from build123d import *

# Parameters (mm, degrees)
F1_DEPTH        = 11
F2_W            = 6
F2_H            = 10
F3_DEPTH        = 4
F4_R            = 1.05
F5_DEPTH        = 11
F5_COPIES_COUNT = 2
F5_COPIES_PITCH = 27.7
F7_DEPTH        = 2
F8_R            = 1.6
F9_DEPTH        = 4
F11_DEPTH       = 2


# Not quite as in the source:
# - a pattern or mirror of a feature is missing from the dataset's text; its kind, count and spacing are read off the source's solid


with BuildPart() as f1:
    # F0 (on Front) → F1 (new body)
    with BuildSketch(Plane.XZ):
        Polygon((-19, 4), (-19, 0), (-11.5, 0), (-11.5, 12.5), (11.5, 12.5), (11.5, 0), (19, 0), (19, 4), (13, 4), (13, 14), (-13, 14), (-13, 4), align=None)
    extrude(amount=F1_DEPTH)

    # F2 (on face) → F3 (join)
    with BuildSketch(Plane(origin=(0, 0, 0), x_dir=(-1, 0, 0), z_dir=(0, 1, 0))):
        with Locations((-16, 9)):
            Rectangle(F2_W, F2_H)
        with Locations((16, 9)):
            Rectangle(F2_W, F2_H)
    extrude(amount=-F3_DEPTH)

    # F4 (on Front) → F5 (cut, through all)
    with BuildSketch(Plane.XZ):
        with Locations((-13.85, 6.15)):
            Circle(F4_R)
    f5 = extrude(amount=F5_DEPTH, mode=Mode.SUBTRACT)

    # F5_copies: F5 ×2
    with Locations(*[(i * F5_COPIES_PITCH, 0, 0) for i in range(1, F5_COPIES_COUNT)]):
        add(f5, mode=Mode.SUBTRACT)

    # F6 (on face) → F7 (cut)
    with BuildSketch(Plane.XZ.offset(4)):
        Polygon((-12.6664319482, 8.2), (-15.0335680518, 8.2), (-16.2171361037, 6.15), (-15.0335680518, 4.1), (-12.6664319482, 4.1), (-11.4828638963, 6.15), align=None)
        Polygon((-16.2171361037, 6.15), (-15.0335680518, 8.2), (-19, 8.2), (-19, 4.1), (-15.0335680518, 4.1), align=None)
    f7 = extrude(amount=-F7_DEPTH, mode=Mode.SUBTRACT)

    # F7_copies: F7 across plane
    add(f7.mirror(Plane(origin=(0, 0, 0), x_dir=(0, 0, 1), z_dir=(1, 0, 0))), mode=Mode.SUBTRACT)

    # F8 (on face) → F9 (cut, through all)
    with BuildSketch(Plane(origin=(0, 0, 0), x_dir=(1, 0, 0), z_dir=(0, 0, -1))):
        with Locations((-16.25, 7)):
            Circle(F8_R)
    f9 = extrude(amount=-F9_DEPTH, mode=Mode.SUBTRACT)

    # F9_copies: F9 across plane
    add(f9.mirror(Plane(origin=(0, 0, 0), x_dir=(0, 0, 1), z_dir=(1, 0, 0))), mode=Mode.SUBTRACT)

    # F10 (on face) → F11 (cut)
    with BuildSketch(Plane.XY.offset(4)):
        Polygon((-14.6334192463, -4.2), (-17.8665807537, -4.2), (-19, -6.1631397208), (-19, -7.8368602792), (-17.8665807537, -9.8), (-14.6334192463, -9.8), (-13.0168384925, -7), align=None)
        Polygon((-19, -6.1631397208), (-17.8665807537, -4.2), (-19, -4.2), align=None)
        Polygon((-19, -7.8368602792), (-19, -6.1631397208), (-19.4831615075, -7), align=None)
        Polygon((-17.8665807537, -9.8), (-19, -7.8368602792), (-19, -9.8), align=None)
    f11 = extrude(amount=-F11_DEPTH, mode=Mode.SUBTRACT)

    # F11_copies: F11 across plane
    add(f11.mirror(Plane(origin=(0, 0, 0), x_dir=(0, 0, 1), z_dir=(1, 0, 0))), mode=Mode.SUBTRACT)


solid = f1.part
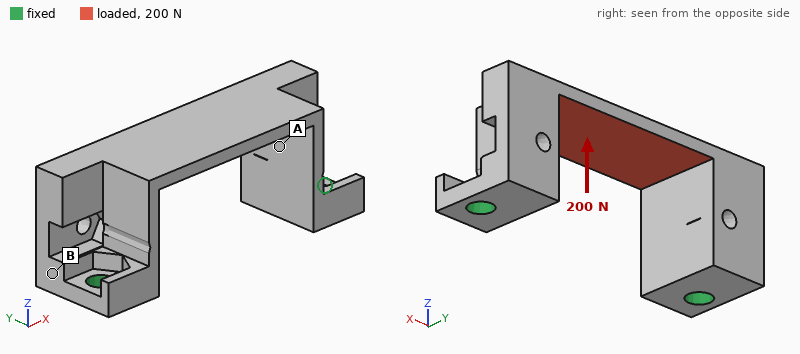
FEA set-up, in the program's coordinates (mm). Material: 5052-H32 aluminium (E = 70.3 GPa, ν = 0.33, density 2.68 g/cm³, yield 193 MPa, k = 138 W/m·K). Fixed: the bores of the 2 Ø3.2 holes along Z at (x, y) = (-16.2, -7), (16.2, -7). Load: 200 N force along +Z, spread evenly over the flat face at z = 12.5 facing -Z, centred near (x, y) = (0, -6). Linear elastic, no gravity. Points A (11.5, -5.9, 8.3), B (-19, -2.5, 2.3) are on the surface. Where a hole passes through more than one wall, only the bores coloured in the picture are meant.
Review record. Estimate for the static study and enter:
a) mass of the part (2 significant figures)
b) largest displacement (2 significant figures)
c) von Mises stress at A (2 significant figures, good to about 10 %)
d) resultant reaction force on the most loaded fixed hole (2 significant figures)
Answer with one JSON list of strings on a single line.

["4.2 g", "52 µm", "20 MPa", "110 N"]
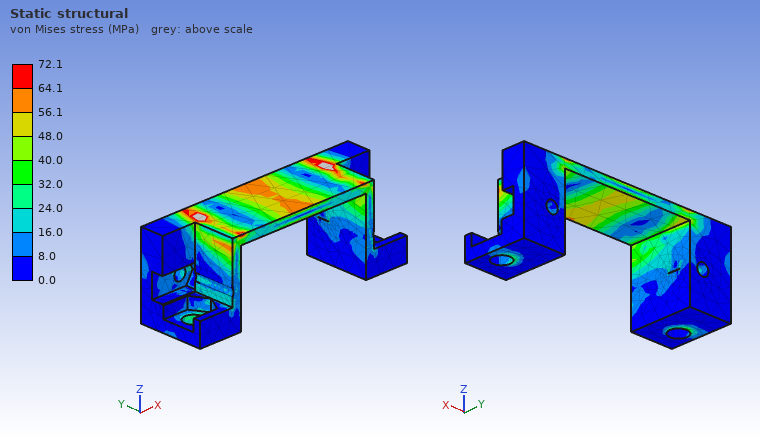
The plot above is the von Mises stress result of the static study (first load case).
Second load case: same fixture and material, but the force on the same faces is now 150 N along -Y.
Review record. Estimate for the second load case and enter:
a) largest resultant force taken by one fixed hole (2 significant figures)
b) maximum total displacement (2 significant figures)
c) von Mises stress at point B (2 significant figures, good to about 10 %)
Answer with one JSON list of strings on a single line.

["77 N", "31 µm", "8.6 MPa"]
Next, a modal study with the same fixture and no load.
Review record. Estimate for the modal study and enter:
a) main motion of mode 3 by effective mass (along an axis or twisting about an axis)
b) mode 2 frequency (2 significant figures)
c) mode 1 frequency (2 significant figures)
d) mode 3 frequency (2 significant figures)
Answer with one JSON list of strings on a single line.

["twisting about Z", "7700 Hz", "7600 Hz", "9300 Hz"]
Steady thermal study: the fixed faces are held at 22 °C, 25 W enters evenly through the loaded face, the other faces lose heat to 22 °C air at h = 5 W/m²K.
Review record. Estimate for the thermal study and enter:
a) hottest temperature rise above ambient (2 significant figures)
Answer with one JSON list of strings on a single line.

["85 K"]
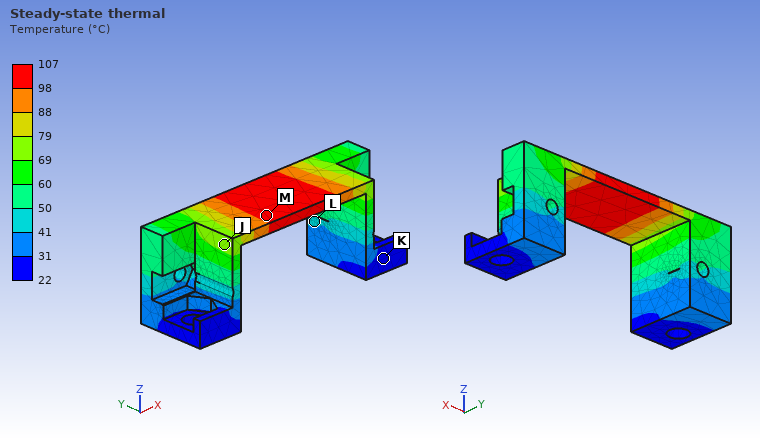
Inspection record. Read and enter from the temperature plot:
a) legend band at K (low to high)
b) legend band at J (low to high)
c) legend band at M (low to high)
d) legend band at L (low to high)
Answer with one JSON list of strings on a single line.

["22 to 31 °C", "69 to 79 °C", "98 to 107 °C", "41 to 50 °C"]
